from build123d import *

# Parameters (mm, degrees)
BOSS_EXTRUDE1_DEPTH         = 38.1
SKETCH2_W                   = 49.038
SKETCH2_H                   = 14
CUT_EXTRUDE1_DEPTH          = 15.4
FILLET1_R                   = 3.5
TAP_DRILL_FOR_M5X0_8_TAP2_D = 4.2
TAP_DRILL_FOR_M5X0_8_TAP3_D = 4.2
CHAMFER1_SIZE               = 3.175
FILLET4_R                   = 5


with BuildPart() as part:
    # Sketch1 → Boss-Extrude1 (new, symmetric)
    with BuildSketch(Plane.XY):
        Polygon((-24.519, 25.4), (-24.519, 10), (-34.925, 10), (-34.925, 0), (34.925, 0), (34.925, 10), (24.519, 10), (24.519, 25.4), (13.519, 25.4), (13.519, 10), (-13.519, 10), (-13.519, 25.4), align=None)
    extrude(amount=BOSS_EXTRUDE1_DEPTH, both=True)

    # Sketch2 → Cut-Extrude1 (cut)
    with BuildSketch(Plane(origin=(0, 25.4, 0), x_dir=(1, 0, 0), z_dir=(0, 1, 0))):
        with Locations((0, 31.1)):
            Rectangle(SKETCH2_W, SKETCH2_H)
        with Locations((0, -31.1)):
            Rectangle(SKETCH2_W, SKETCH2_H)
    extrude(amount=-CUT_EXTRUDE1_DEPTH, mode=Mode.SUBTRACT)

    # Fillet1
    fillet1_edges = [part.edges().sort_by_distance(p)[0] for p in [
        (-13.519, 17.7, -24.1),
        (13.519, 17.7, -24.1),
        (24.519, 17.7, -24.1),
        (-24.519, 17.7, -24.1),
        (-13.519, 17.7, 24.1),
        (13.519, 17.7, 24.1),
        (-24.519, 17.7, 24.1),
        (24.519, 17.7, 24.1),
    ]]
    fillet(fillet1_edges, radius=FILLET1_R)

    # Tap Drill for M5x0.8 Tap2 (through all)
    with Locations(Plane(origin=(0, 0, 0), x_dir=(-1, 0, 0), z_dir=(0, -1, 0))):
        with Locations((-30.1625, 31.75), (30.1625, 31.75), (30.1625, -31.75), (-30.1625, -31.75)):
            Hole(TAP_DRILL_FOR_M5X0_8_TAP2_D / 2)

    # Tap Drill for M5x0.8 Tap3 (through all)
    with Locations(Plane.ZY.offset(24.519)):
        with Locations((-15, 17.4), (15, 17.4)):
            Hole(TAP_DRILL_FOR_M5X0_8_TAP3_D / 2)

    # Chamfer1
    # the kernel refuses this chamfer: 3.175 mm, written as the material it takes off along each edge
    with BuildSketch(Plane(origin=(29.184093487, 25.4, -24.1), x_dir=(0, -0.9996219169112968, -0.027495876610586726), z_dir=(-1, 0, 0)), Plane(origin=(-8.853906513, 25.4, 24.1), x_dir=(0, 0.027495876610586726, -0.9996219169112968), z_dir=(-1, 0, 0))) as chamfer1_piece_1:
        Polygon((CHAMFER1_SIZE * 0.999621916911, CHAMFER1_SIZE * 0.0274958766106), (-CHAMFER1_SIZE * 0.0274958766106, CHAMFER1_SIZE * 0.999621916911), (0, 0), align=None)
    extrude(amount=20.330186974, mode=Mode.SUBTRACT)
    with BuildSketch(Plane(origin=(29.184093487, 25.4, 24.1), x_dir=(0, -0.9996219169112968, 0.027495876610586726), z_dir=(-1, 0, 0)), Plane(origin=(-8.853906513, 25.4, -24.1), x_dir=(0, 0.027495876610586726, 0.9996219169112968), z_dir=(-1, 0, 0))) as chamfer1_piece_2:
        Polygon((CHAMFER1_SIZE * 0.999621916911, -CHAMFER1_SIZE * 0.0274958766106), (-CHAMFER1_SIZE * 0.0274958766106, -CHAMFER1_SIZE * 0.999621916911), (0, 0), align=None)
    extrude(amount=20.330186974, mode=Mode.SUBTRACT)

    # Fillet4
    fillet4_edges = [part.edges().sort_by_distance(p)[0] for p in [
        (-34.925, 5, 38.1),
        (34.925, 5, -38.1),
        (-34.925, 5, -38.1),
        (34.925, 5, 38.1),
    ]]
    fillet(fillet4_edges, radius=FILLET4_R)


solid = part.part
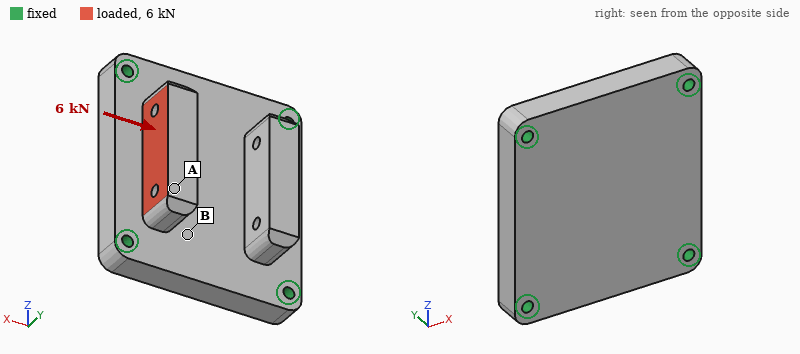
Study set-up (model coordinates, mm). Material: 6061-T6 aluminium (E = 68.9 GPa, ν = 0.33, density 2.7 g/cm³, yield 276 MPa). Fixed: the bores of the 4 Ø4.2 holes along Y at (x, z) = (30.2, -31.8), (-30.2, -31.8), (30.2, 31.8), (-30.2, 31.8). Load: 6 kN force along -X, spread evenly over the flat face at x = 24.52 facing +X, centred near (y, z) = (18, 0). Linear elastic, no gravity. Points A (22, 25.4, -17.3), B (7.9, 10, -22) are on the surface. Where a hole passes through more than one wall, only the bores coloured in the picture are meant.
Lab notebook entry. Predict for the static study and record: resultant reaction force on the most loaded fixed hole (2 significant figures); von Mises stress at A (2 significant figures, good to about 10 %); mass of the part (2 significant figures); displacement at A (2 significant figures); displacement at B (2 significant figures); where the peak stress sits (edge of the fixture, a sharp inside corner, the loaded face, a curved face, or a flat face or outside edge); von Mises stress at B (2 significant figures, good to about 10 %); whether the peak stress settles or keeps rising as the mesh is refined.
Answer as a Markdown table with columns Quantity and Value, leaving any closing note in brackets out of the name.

| Quantity | Value |
|---|---|
| resultant reaction force on the most loaded fixed hole | 2.0 kN |
| von Mises stress at A | 11 MPa |
| mass of the part | 180 g |
| displacement at A | 50 µm |
| displacement at B | 14 µm |
| where the peak stress sits | edge of the fixture |
| von Mises stress at B | 27 MPa |
| whether the peak stress settles or keeps rising as the mesh is refined | keeps rising |
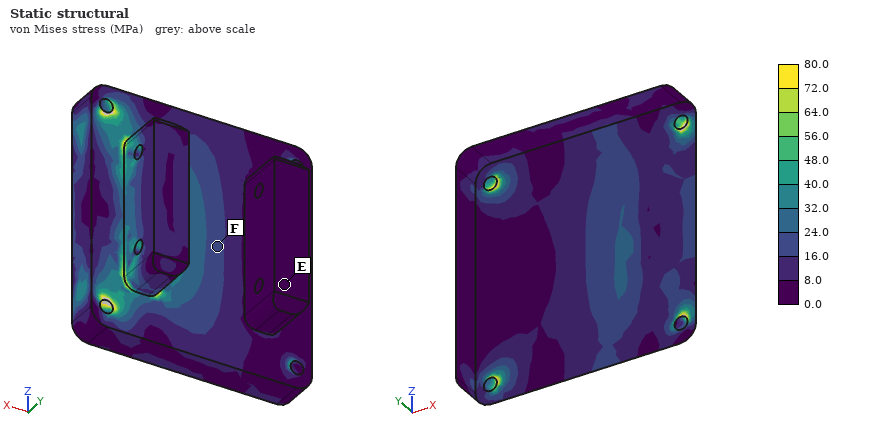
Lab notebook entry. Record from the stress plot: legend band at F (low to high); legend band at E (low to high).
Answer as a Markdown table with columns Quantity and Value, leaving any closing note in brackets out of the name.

| Quantity | Value |
|---|---|
| legend band at F | 16.0 to 24.0 MPa |
| legend band at E | 0.0 to 8.0 MPa |
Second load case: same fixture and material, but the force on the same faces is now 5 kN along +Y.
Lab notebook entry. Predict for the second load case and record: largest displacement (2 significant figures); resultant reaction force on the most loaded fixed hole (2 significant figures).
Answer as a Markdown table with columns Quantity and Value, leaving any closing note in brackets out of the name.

| Quantity | Value |
|---|---|
| largest displacement | 35 µm |
| resultant reaction force on the most loaded fixed hole | 2.4 kN |
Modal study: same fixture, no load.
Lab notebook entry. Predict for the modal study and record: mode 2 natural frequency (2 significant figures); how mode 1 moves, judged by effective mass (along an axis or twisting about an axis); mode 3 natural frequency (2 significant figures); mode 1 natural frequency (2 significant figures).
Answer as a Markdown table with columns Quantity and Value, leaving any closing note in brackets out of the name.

| Quantity | Value |
|---|---|
| mode 2 natural frequency | 11 kHz |
| how mode 1 moves, judged by effective mass | along Y |
| mode 3 natural frequency | 12 kHz |
| mode 1 natural frequency | 7100 Hz |
